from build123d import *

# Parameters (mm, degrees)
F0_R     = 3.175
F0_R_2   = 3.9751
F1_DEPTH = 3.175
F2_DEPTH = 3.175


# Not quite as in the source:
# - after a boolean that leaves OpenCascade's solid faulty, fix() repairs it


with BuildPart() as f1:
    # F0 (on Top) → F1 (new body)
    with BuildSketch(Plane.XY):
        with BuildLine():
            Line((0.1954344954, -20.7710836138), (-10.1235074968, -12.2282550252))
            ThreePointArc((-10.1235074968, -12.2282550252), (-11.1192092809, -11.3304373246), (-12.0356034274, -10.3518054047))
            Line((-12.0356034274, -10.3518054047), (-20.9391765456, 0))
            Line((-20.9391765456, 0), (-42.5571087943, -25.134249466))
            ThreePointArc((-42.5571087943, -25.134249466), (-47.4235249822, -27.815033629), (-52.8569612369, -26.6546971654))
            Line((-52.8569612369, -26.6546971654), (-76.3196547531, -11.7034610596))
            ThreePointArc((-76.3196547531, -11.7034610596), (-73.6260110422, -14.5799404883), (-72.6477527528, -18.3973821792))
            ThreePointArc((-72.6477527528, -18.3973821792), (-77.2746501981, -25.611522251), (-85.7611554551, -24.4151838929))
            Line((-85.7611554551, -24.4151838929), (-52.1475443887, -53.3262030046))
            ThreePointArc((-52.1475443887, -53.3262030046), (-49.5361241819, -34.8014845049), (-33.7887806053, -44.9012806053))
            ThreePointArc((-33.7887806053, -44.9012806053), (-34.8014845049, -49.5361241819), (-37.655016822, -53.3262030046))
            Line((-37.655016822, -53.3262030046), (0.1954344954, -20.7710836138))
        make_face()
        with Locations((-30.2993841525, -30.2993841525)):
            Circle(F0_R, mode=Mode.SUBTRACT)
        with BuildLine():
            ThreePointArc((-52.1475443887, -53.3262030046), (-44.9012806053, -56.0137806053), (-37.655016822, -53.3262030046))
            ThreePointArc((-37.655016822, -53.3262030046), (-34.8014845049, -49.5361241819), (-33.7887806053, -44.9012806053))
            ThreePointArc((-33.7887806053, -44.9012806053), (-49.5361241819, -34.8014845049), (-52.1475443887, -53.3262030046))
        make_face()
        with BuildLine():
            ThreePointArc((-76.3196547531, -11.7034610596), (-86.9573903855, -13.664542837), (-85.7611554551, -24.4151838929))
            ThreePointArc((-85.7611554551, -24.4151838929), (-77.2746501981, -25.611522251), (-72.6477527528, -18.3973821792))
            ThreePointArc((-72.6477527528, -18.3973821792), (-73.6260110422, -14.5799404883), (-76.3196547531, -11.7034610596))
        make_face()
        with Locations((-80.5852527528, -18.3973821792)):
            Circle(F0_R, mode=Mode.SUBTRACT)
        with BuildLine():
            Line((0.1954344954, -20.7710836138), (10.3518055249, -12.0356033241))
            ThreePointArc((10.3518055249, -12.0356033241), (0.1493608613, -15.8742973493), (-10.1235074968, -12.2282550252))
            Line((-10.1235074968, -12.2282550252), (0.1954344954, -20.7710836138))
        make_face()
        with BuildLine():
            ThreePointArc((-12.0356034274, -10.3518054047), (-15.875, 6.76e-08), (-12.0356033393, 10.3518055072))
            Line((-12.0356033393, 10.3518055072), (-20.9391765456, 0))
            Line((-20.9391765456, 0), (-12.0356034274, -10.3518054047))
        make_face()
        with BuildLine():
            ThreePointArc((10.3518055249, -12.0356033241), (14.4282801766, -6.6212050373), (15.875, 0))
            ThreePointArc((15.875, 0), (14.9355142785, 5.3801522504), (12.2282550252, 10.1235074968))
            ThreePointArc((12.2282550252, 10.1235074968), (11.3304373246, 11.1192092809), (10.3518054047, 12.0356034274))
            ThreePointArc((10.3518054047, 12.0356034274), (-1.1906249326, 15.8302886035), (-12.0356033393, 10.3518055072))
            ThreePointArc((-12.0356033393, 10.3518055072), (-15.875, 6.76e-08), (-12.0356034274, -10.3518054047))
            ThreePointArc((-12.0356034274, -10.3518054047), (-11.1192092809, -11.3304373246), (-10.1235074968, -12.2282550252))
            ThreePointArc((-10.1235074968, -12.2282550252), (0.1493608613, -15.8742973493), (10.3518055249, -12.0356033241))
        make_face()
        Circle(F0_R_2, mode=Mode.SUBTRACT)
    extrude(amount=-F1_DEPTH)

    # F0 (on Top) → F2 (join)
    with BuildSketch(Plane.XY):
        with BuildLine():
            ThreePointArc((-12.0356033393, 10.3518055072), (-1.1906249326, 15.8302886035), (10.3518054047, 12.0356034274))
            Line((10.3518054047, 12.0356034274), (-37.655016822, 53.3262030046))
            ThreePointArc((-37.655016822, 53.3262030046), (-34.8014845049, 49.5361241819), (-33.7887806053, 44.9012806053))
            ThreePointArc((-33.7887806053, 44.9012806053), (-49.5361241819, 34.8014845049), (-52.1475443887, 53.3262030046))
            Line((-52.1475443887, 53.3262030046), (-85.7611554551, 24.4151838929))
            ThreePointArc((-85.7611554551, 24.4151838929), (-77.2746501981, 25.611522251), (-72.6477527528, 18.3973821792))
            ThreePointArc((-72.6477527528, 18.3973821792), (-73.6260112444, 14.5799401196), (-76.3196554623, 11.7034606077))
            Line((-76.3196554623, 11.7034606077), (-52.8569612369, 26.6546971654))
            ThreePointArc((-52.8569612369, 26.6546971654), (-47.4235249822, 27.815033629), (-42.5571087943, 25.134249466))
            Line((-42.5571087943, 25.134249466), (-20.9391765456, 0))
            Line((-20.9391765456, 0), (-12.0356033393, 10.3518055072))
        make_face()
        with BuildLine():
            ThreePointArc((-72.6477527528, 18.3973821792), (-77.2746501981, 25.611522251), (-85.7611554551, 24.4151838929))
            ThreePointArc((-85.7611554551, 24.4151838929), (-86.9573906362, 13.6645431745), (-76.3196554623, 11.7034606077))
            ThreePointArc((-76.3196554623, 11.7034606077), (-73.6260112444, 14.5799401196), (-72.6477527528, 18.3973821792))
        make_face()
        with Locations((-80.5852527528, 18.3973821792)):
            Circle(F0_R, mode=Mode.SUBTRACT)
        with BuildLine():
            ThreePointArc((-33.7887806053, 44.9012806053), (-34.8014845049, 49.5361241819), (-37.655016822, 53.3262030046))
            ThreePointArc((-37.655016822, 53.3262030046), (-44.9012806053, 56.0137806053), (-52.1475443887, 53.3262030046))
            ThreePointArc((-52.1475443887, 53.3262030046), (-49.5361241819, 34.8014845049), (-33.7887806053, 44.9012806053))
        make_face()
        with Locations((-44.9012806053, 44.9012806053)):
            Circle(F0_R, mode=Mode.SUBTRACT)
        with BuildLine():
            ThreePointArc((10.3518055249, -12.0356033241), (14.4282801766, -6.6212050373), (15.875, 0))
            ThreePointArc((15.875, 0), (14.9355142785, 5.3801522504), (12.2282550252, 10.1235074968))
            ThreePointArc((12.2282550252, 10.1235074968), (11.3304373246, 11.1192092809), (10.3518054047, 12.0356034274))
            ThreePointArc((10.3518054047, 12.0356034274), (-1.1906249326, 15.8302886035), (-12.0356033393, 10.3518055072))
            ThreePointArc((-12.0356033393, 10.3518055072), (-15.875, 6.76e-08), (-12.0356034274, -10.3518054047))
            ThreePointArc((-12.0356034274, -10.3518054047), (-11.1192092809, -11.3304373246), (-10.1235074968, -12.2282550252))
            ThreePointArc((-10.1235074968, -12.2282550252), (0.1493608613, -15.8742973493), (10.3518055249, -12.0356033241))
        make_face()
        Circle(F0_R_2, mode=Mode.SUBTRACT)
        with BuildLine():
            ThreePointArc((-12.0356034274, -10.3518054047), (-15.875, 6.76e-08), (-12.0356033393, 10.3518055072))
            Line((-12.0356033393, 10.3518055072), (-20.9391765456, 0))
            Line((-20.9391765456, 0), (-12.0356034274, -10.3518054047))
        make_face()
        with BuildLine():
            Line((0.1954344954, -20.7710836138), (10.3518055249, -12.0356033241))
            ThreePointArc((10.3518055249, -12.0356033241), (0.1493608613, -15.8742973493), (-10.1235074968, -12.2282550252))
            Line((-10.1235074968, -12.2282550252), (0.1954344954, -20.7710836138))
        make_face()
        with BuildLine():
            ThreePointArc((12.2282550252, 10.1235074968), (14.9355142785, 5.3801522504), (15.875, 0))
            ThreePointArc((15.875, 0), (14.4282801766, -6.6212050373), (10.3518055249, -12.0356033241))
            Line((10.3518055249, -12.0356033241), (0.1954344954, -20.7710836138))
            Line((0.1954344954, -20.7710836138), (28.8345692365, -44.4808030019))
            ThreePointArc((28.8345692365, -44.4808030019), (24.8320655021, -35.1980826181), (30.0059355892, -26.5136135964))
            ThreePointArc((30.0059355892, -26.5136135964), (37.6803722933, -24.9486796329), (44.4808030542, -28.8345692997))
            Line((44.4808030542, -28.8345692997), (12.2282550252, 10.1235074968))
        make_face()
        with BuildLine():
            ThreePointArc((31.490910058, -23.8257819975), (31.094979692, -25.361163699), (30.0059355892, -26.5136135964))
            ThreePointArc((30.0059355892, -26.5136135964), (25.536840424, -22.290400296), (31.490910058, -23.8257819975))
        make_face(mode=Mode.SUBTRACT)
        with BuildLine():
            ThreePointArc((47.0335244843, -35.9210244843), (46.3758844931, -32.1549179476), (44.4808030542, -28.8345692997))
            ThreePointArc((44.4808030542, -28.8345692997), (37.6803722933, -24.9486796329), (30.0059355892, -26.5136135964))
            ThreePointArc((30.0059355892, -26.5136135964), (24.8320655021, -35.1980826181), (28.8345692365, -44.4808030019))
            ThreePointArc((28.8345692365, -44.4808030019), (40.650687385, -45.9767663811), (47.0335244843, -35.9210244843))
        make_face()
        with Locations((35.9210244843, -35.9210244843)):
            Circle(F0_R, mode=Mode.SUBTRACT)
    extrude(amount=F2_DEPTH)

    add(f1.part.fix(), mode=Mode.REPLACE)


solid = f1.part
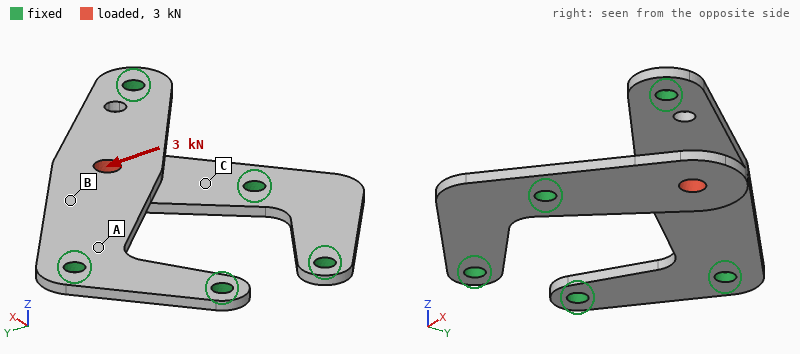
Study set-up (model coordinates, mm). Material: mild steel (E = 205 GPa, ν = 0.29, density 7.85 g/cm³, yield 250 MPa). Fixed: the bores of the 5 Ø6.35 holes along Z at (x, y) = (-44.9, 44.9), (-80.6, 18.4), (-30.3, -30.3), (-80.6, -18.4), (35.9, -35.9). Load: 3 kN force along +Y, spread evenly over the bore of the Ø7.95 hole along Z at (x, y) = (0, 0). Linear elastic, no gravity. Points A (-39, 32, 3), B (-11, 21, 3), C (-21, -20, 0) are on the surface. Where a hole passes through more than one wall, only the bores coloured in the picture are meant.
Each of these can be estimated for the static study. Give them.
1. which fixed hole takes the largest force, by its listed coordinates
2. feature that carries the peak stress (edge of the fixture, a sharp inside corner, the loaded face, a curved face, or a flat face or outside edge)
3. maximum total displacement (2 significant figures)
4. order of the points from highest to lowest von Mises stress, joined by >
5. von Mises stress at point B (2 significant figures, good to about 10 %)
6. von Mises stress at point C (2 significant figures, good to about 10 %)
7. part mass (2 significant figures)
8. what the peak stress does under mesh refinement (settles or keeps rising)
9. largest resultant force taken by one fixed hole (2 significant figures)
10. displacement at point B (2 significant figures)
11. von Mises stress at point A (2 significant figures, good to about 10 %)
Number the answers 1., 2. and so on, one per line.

1. (-30.3, -30.3)
2. edge of the fixture
3. 18 µm
4. C > A > B
5. 7.0 MPa
6. 31 MPa
7. 170 g
8. keeps rising
9. 1.8 kN
10. 6.5 µm
11. 14 MPa
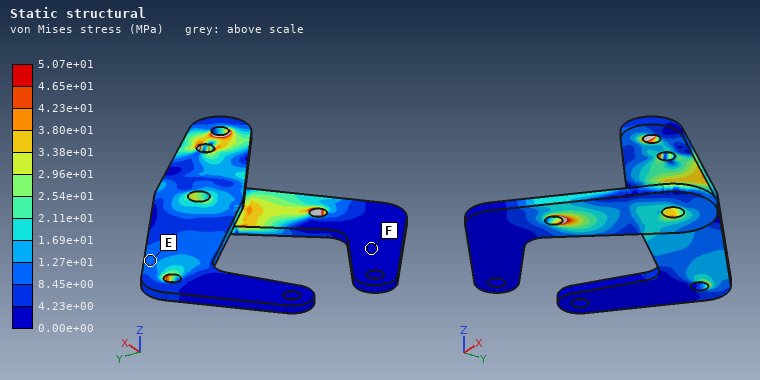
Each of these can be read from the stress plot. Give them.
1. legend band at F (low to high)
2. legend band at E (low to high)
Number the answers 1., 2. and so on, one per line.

1. 0.00e+00 to 4.23e+00 MPa
2. 8.45e+00 to 1.27e+01 MPa
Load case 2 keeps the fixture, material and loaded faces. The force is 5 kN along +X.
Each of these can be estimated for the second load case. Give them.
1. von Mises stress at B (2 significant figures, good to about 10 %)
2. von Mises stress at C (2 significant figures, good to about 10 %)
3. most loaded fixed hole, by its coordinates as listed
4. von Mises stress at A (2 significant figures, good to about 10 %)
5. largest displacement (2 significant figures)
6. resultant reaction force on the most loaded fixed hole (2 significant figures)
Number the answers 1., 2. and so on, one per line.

1. 11 MPa
2. 53 MPa
3. (-30.3, -30.3)
4. 41 MPa
5. 46 µm
6. 2.8 kN
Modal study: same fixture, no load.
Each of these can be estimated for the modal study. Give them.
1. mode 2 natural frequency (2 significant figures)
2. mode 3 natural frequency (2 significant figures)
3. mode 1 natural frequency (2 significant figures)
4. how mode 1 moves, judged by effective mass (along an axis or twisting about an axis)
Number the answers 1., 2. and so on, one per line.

1. 3700 Hz
2. 3900 Hz
3. 1600 Hz
4. along Z
